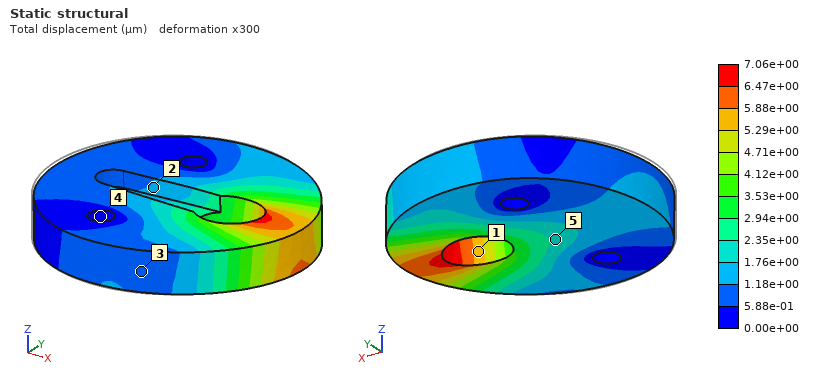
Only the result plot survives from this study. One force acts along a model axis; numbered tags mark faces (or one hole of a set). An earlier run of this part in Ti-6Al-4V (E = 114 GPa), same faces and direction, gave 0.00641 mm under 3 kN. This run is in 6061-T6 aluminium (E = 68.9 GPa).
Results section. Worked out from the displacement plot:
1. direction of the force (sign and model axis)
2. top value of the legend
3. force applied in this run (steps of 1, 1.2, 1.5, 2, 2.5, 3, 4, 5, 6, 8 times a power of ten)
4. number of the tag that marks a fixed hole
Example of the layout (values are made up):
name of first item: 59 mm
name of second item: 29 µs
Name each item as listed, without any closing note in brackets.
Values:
direction of the force: +X
top value of the legend: 7.06e+00 µm
force applied in this run: 2 kN
number of the tag that marks a fixed hole: 4
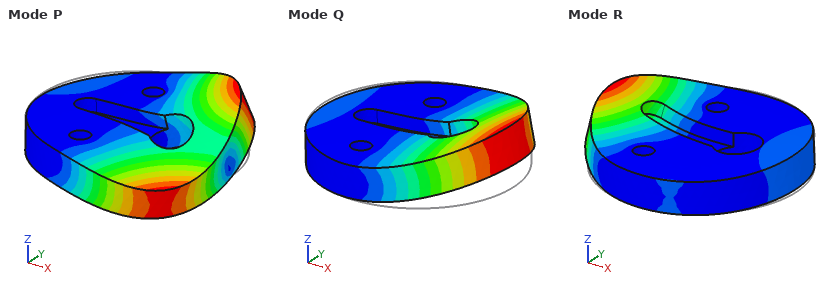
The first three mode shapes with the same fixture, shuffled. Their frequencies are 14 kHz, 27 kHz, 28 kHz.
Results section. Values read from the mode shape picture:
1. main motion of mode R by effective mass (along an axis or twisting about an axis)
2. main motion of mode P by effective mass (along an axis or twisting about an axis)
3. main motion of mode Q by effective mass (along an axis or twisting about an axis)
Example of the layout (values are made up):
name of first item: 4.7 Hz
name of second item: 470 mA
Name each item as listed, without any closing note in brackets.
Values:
main motion of mode R by effective mass: along Z
main motion of mode P by effective mass: twisting about X
main motion of mode Q by effective mass: along Z
